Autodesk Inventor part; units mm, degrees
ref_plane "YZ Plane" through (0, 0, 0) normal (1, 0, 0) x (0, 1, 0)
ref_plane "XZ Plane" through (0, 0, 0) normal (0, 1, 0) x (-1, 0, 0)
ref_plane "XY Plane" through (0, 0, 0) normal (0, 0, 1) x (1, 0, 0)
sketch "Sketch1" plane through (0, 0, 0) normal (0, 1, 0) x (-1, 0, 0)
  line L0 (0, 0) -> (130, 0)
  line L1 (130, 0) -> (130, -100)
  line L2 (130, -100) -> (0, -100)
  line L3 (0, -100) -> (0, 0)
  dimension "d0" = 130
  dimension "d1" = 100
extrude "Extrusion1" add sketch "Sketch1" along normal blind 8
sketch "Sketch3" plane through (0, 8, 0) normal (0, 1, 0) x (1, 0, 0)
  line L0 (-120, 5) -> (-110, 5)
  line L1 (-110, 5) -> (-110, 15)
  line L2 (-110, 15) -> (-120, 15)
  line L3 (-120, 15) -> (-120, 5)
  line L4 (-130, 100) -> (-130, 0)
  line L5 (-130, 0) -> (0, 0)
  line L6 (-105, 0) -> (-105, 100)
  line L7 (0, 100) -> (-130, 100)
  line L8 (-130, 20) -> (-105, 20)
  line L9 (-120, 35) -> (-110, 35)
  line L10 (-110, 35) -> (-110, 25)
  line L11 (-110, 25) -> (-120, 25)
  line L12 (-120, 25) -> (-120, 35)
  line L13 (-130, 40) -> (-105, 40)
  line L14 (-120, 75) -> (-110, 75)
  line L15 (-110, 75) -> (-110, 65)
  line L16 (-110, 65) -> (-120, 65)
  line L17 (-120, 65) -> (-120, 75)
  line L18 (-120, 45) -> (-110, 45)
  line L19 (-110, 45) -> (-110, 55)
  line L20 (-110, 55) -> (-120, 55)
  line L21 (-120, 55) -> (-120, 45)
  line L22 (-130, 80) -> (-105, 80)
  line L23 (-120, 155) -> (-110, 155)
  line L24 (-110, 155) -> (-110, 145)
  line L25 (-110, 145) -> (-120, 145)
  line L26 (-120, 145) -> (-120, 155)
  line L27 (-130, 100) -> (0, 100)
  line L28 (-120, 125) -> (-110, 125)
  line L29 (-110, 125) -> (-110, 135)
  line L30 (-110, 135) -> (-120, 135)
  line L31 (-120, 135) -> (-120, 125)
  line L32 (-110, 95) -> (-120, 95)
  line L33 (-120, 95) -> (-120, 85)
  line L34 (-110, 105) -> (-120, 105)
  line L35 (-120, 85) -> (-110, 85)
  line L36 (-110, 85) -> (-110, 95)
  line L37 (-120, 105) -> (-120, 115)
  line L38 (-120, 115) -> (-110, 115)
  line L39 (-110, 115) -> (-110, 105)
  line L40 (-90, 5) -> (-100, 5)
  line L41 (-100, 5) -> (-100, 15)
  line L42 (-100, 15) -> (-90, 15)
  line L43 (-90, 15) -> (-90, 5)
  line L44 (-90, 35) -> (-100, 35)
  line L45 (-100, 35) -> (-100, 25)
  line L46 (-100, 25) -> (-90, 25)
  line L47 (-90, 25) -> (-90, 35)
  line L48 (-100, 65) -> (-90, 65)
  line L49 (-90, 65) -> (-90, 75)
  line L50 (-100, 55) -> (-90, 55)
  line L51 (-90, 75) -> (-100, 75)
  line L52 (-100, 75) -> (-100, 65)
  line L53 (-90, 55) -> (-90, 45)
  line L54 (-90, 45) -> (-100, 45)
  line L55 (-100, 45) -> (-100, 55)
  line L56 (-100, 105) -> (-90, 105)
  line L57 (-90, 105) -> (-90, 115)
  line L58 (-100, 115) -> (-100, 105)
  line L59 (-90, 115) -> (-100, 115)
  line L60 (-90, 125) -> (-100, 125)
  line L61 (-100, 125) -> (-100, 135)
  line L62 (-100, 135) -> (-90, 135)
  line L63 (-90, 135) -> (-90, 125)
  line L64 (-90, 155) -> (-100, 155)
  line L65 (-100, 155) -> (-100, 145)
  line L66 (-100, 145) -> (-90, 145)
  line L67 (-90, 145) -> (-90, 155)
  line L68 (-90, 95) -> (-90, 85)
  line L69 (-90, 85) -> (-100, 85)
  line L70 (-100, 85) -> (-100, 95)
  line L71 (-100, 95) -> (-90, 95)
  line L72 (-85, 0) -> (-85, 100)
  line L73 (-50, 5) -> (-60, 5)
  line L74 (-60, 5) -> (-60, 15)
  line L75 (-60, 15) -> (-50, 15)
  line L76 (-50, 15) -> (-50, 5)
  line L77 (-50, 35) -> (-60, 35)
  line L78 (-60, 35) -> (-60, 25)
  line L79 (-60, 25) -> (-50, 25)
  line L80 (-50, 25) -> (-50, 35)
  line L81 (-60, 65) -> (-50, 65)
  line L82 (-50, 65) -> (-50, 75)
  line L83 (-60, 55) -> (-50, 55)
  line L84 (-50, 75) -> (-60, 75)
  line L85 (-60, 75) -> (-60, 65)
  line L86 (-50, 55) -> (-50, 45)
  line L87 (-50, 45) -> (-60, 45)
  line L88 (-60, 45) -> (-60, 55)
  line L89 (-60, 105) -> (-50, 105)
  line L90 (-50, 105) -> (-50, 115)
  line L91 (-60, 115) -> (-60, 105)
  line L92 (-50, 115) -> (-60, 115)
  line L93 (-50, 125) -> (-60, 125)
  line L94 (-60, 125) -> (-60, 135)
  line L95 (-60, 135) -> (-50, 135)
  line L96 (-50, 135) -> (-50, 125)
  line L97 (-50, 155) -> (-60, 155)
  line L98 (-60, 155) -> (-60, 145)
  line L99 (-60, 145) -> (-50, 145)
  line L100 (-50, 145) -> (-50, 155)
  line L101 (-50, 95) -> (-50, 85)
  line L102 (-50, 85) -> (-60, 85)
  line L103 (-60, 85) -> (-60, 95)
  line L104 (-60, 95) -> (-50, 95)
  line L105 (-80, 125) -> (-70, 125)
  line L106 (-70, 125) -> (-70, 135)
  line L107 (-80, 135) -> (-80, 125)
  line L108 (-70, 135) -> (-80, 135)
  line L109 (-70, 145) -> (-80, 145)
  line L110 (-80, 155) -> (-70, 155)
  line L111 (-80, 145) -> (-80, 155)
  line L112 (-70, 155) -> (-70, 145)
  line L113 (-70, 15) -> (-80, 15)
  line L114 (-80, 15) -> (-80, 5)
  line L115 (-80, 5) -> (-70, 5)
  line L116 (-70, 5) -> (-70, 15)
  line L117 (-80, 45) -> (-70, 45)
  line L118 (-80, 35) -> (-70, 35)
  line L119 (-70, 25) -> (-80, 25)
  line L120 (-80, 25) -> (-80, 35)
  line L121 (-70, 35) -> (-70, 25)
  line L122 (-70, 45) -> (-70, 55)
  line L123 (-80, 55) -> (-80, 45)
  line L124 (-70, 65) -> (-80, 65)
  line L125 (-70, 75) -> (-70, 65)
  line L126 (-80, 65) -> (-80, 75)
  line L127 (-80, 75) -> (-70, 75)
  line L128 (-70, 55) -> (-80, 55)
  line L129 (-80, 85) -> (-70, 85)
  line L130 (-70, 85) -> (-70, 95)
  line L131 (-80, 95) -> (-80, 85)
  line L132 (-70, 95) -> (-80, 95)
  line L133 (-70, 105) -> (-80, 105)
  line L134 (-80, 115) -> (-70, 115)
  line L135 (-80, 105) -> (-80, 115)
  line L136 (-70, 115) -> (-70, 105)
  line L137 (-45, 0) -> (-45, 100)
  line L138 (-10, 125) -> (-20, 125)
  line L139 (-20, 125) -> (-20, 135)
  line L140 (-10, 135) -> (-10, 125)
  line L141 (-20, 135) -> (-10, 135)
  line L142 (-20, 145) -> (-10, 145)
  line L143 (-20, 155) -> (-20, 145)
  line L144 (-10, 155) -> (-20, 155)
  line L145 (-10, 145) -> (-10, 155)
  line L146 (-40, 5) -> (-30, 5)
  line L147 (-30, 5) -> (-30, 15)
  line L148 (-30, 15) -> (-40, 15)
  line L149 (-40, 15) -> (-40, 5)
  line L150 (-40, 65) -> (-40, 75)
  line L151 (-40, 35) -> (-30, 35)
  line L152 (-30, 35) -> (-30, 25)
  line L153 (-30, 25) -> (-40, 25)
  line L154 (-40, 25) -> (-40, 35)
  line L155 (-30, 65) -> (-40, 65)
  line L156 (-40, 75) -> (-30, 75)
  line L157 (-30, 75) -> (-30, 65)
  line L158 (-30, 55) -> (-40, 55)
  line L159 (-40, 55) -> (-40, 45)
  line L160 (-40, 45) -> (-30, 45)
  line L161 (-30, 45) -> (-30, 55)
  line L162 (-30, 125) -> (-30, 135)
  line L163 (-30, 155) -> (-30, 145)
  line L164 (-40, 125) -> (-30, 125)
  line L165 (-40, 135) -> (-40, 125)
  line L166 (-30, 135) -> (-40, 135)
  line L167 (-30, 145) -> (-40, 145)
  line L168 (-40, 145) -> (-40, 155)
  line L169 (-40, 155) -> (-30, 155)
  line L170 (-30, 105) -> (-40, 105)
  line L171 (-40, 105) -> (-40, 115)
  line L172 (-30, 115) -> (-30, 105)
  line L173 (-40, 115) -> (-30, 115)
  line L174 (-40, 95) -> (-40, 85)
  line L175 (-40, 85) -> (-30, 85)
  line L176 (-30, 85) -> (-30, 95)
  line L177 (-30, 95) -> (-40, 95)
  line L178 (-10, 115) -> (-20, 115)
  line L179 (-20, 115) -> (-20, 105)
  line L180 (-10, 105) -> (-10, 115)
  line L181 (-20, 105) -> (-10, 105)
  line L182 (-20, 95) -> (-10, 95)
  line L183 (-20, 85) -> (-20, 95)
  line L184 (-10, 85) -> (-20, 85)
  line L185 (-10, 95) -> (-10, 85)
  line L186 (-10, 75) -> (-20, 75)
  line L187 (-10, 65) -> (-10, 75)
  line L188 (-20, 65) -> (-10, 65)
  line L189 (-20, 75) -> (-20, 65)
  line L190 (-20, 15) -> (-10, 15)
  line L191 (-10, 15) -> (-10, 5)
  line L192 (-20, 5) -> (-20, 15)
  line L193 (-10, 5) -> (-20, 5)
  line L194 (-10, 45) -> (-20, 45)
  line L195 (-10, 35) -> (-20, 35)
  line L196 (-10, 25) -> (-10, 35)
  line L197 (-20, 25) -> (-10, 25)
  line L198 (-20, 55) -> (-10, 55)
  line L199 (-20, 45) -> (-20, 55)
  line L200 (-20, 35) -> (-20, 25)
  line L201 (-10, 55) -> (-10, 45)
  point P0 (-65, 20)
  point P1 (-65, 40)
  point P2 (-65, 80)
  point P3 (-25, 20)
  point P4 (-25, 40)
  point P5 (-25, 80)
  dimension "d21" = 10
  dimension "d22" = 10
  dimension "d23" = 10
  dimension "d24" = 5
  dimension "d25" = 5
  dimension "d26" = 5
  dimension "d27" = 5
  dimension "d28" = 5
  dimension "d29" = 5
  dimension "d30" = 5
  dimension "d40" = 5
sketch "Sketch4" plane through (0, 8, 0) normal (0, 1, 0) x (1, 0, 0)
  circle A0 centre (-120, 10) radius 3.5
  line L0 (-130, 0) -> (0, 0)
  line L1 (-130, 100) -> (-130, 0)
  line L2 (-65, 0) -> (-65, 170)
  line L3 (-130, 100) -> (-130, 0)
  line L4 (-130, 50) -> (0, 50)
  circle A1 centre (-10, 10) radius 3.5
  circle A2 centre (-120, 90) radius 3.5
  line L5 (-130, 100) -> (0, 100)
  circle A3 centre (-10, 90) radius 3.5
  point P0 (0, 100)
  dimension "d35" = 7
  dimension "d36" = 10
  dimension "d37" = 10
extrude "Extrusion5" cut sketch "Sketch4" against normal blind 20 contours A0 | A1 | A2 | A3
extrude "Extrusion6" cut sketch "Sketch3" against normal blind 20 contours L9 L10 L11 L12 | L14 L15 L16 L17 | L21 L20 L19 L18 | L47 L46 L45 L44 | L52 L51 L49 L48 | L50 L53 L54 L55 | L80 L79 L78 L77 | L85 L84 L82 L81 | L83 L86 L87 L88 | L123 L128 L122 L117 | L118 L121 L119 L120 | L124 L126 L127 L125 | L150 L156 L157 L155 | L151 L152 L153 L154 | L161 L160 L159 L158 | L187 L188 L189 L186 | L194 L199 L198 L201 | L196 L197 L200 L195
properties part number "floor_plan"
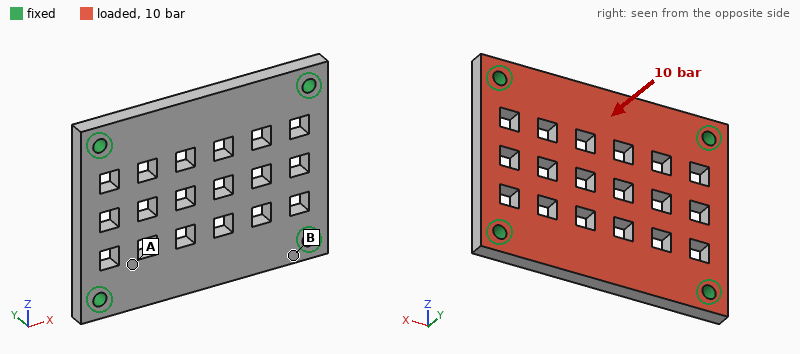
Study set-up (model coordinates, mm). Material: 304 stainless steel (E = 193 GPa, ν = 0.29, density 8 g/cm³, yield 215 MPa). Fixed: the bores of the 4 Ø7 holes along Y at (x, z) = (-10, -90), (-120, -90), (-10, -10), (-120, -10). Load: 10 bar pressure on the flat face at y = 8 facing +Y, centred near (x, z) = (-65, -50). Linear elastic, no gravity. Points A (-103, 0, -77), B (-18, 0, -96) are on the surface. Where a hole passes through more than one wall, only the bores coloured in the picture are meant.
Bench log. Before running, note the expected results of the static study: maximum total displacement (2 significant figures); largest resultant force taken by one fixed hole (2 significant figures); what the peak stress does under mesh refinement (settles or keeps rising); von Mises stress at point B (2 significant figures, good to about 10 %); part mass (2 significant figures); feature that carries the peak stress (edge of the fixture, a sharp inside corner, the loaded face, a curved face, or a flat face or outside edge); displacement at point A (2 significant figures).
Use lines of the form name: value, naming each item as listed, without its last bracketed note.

maximum total displacement: 84 µm
largest resultant force taken by one fixed hole: 2.8 kN
what the peak stress does under mesh refinement: keeps rising
von Mises stress at point B: 77 MPa
part mass: 710 g
feature that carries the peak stress: edge of the fixture
displacement at point A: 30 µm
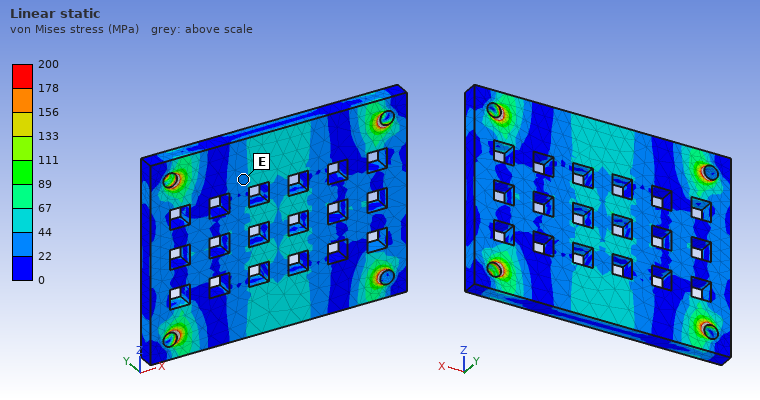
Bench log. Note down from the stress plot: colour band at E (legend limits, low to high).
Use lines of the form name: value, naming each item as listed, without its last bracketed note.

colour band at E: 22 to 44 MPa
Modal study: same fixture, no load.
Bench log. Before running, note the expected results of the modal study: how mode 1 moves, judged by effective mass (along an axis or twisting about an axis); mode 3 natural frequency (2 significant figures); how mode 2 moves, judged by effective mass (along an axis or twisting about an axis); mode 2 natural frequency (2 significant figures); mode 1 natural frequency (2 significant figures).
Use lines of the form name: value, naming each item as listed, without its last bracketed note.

how mode 1 moves, judged by effective mass: along Y
mode 3 natural frequency: 5300 Hz
how mode 2 moves, judged by effective mass: twisting about X
mode 2 natural frequency: 3800 Hz
mode 1 natural frequency: 2600 Hz
